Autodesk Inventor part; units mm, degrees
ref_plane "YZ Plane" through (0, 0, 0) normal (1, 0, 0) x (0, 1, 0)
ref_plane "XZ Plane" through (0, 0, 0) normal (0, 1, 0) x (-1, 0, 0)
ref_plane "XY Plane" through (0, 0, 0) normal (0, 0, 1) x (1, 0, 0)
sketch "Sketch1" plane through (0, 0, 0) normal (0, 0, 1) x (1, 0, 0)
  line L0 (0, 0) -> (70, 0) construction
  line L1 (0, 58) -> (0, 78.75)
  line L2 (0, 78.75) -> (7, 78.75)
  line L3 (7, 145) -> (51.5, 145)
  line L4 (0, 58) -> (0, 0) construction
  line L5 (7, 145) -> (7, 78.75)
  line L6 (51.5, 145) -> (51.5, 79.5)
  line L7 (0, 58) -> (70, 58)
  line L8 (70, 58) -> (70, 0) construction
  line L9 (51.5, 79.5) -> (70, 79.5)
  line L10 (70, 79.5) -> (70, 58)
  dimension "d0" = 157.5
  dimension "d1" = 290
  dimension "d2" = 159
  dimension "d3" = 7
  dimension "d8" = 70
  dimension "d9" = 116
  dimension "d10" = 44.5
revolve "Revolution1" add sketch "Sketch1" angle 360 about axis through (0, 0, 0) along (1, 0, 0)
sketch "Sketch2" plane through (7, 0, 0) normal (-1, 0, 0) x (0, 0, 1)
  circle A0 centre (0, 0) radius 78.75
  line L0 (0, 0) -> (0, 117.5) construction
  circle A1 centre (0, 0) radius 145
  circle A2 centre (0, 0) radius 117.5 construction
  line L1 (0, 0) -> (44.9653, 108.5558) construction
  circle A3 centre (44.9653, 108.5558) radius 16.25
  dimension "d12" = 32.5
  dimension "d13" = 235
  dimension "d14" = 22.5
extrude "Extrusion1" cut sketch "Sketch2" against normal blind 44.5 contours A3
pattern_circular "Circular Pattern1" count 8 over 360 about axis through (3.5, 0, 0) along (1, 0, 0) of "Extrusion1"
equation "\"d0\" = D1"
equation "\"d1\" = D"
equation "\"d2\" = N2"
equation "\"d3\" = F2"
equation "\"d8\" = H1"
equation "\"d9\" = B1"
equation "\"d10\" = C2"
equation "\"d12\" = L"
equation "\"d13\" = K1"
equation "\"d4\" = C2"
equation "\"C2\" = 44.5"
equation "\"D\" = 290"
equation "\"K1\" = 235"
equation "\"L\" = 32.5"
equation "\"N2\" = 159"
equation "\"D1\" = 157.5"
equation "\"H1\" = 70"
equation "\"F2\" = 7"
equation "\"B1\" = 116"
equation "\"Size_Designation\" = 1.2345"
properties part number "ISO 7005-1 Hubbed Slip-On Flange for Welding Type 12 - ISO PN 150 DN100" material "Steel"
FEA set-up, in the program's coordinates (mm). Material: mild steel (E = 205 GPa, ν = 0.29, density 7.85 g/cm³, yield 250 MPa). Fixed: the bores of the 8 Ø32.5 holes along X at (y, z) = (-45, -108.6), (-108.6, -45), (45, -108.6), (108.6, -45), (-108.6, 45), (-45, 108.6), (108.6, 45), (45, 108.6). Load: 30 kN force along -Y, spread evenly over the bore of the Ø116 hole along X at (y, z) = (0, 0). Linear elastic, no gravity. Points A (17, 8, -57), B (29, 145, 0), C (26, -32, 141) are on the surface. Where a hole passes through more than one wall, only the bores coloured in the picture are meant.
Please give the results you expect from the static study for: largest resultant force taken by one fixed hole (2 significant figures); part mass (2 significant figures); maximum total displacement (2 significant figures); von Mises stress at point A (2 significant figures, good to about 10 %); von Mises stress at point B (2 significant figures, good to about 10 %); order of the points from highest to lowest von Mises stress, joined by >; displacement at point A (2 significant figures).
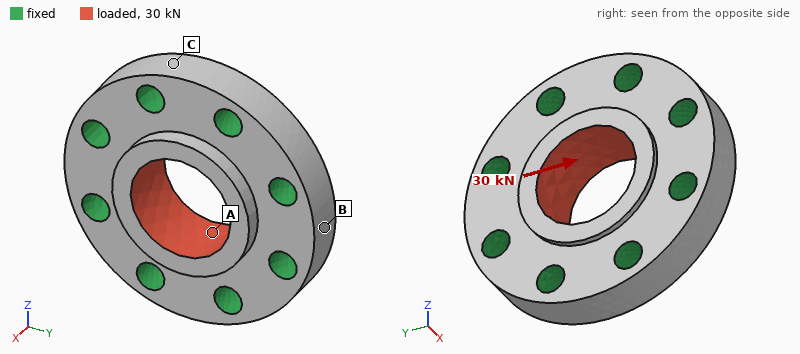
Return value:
5.3 kN
19 kg
1.1 µm
2.1 MPa
0.62 MPa
A > B > C
0.46 µm
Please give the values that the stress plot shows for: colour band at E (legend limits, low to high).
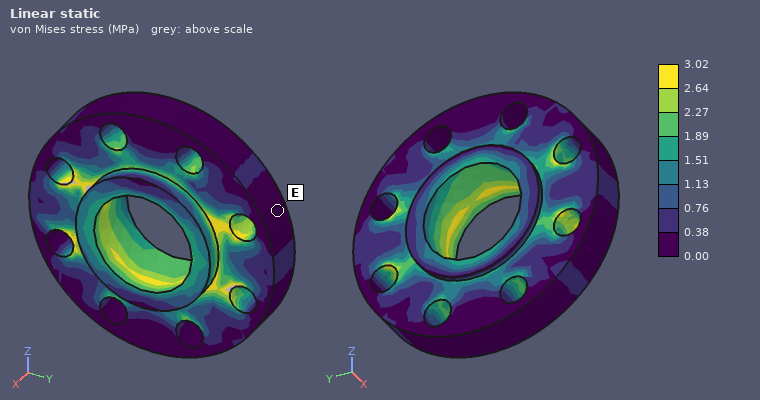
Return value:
0.00 to 0.38 MPa
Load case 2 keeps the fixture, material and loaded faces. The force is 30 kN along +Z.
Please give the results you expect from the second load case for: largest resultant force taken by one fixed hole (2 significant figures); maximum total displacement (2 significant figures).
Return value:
5.3 kN
1.1 µm
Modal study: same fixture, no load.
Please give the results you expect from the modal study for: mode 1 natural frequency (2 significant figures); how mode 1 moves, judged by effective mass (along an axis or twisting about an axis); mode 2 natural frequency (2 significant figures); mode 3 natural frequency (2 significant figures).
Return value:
9600 Hz
along X
11 kHz
11 kHz
